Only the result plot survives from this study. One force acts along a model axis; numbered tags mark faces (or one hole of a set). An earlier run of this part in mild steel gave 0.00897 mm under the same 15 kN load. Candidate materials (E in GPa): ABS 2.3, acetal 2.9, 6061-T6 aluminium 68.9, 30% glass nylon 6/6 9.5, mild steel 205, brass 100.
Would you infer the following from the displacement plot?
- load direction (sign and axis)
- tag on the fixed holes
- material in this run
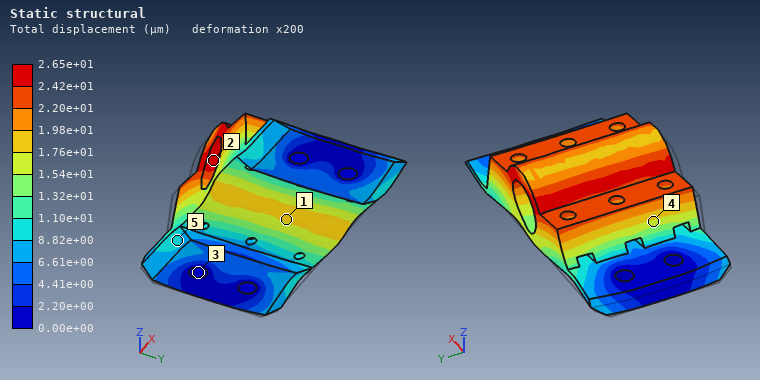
+X
3
6061-T6 aluminium
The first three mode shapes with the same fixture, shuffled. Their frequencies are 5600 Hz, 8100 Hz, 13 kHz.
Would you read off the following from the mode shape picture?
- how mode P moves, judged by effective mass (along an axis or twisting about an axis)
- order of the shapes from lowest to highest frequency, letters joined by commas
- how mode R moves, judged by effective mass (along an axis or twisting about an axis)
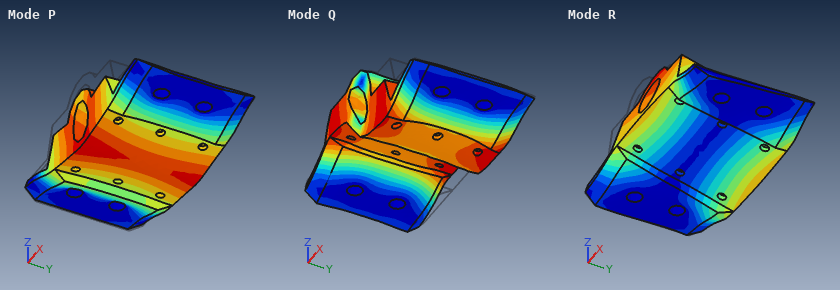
along Z
R, P, Q
along Y
